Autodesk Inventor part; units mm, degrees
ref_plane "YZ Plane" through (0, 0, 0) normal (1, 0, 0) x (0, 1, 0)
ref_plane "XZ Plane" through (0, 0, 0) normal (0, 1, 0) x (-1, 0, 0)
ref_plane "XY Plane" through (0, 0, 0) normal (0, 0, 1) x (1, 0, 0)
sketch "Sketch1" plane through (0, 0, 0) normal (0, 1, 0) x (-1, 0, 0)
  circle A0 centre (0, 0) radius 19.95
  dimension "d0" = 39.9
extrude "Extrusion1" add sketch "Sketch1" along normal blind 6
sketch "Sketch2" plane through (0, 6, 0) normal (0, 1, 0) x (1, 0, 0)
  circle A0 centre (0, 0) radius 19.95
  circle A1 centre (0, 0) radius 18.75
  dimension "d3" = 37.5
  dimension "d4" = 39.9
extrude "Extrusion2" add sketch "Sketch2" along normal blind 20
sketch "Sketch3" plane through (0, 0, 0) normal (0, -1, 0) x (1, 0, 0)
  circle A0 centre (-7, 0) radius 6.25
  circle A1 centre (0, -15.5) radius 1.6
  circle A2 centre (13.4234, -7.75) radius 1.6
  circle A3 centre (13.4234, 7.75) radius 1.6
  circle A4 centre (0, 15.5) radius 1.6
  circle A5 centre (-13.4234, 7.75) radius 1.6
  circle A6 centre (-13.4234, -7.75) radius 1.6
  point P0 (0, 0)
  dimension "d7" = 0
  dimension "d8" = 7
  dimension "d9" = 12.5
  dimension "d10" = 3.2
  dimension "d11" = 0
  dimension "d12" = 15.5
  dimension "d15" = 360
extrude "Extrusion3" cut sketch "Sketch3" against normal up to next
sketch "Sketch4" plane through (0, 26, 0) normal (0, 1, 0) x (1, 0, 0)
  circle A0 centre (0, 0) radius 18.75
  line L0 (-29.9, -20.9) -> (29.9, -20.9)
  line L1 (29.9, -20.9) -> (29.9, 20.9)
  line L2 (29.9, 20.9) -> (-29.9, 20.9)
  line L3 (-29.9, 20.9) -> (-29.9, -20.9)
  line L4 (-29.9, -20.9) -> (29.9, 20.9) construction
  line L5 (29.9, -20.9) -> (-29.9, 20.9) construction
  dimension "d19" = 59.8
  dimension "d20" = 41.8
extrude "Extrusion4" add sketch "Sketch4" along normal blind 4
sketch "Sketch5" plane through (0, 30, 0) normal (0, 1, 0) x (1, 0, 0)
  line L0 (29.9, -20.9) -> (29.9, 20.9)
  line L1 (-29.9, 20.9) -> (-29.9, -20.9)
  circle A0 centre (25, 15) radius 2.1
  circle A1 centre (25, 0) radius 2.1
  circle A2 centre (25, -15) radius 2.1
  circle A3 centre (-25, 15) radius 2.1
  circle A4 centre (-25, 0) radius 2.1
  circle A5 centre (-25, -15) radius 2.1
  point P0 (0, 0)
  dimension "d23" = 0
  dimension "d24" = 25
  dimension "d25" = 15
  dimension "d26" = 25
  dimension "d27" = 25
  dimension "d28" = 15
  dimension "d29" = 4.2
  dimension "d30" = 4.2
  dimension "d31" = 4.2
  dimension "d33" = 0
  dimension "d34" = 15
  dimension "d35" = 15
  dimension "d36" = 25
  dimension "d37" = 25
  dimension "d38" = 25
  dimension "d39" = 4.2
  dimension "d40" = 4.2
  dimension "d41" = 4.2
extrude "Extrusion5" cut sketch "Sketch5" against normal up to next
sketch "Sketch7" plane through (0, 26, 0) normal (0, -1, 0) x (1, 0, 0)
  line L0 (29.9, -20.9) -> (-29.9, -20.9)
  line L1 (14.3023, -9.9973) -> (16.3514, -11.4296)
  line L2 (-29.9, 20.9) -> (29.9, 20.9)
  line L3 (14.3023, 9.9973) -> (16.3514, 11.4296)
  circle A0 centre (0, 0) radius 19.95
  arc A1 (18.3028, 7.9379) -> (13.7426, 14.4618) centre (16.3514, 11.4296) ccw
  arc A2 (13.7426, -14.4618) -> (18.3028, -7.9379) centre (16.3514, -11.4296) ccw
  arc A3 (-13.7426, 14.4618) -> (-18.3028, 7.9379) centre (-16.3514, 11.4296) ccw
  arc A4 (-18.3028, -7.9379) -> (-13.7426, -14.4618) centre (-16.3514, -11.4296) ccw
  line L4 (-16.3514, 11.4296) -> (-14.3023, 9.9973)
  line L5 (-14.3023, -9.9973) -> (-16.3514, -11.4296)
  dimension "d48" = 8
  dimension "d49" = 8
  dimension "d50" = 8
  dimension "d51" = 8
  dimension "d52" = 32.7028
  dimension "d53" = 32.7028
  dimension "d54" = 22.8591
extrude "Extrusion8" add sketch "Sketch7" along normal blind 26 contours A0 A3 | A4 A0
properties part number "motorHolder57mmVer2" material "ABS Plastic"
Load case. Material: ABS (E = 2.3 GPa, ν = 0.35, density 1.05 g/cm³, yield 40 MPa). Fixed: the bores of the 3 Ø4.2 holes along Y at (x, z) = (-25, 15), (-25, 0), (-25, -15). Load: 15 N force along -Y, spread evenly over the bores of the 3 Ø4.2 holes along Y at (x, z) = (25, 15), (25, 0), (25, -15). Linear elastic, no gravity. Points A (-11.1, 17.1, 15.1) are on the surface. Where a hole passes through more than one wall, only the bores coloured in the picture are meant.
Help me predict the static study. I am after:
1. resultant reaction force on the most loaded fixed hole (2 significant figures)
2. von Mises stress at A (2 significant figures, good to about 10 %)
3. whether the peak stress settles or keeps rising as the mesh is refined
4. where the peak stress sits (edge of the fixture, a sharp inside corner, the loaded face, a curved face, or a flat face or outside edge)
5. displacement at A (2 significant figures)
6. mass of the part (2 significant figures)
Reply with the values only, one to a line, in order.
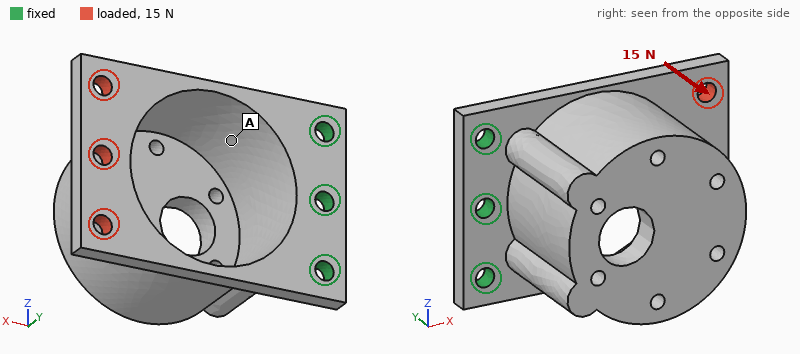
12 N
1.5 MPa
keeps rising
edge of the fixture
0.20 mm
17 g
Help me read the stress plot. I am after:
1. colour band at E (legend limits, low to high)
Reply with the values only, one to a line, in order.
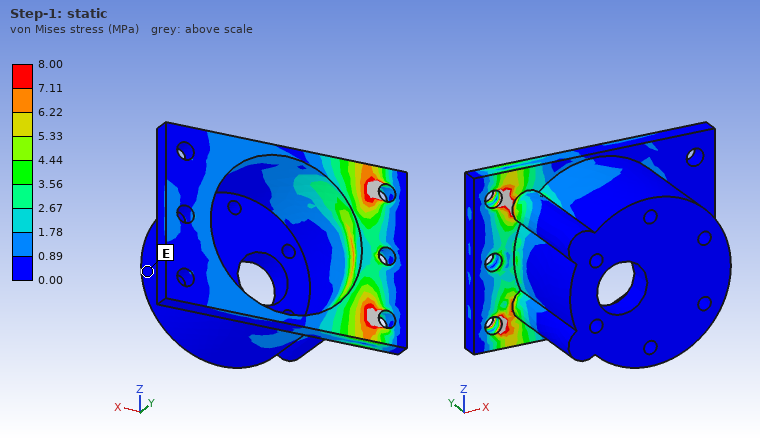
0.00 to 0.89 MPa
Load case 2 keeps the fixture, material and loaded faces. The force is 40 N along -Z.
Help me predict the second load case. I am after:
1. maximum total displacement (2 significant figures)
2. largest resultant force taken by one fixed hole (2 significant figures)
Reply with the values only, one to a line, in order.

0.61 mm
57 N
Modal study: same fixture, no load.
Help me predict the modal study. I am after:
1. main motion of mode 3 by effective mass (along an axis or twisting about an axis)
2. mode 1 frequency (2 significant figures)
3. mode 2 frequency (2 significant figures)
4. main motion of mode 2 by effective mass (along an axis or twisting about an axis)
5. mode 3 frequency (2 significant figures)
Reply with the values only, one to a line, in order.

along Z
270 Hz
620 Hz
along Z
1300 Hz
